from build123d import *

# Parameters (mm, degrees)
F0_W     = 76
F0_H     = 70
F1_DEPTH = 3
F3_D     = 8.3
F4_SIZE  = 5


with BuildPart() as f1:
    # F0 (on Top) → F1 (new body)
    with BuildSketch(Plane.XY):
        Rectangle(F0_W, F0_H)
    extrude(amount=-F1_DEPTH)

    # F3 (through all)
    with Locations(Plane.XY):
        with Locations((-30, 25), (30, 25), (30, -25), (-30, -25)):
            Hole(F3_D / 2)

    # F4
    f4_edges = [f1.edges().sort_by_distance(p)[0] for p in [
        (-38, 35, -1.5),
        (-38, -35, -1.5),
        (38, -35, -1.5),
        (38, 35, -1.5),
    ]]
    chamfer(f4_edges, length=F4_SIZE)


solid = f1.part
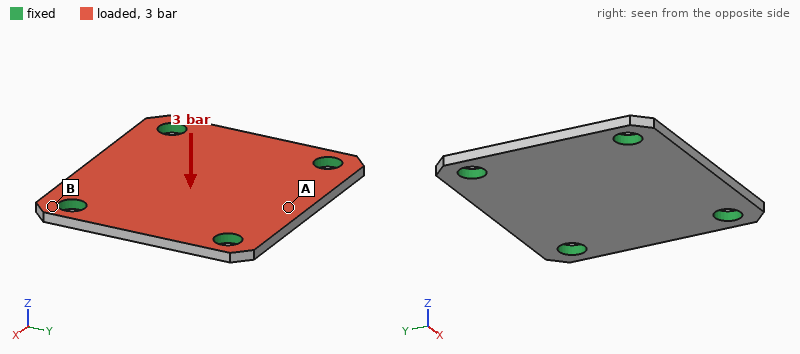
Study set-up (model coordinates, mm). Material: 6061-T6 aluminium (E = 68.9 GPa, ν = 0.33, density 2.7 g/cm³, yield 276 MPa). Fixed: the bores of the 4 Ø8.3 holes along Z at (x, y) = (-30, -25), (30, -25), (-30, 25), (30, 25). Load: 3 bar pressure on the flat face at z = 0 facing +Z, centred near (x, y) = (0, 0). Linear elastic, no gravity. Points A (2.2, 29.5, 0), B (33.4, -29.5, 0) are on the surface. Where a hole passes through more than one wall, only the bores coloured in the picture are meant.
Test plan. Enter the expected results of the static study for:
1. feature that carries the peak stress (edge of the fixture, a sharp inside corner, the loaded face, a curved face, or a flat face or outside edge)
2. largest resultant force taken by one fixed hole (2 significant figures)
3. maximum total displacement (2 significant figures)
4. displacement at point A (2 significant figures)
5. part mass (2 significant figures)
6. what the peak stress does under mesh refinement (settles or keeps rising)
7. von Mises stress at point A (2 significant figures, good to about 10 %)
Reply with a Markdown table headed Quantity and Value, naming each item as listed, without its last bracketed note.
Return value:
| Quantity | Value |
|---|---|
| feature that carries the peak stress | edge of the fixture |
| largest resultant force taken by one fixed hole | 380 N |
| maximum total displacement | 79 µm |
| displacement at point A | 50 µm |
| part mass | 41 g |
| what the peak stress does under mesh refinement | keeps rising |
| von Mises stress at point A | 27 MPa |
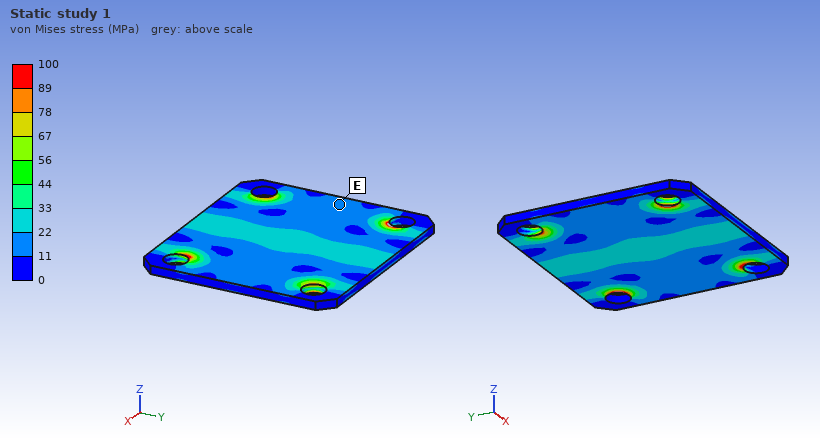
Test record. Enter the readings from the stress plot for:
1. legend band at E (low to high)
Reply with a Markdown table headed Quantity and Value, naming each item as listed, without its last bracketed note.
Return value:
| Quantity | Value |
|---|---|
| legend band at E | 11 to 22 MPa |
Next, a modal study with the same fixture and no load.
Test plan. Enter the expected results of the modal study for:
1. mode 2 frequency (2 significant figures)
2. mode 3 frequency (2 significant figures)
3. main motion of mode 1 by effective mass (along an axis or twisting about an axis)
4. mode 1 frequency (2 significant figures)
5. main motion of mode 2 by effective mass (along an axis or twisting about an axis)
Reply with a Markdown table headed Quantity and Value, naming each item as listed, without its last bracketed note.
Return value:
| Quantity | Value |
|---|---|
| mode 2 frequency | 5800 Hz |
| mode 3 frequency | 6800 Hz |
| main motion of mode 1 by effective mass | along Z |
| mode 1 frequency | 4200 Hz |
| main motion of mode 2 by effective mass | twisting about X |
